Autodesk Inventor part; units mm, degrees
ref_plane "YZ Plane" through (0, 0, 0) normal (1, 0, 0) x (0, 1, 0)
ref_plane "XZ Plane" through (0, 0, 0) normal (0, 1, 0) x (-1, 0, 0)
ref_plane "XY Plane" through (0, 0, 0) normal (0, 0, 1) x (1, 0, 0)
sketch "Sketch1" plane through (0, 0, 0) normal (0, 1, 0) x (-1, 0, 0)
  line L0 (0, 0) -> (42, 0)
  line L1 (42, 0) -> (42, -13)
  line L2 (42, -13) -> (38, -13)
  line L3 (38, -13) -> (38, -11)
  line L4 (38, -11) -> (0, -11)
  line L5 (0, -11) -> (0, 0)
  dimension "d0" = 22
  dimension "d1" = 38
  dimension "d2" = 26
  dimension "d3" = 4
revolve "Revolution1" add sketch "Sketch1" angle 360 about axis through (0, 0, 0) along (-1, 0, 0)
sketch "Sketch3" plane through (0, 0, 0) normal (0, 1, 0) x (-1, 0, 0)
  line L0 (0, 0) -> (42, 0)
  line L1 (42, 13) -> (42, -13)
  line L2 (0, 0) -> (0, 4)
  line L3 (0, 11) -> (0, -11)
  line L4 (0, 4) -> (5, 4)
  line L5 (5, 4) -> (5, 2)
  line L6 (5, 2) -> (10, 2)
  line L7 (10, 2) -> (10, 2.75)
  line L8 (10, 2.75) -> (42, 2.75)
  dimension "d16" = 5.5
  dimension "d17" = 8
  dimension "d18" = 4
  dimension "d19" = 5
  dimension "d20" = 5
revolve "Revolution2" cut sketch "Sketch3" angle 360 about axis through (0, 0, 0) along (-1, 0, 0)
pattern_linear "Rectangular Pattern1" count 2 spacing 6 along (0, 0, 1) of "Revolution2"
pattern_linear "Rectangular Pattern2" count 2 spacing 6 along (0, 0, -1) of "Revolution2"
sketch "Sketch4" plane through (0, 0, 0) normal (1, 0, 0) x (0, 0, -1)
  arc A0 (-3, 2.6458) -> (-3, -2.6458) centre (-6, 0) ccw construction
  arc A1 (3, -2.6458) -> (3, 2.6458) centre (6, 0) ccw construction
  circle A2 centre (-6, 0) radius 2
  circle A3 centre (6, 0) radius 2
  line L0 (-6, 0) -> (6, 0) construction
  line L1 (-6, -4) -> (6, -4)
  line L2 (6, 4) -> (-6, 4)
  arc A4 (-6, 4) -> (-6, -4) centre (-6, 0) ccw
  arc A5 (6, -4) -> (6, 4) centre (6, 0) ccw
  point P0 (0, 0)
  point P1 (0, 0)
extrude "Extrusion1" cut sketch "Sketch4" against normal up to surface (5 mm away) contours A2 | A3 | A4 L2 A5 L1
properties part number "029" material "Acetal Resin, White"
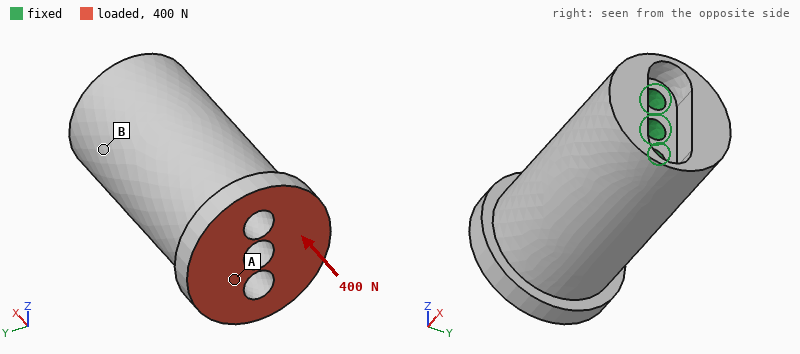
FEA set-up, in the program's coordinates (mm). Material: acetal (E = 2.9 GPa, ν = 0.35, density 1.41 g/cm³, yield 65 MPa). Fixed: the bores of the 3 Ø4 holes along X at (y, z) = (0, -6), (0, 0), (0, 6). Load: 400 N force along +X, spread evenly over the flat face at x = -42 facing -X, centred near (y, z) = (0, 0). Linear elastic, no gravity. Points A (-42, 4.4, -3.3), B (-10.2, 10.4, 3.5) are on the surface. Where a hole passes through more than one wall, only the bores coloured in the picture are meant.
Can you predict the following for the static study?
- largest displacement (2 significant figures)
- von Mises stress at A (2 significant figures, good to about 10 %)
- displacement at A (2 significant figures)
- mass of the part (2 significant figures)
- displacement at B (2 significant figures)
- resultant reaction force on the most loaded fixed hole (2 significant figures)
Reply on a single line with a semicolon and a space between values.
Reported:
23 µm; 1.4 MPa; 19 µm; 19 g; 9.2 µm; 140 N
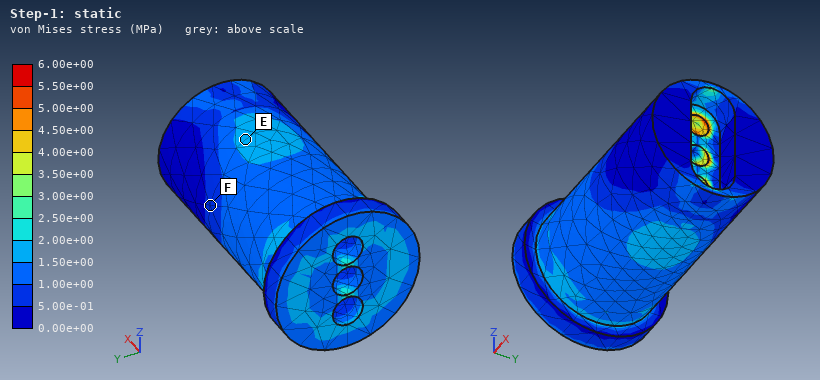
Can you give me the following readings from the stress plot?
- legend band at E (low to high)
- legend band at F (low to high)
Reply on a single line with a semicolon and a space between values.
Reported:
1.50e+00 to 2.00e+00 MPa; 5.00e-01 to 1.00e+00 MPa
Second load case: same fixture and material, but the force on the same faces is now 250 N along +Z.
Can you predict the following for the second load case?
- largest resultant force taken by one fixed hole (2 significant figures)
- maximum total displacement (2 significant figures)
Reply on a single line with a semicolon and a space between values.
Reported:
540 N; 0.25 mm
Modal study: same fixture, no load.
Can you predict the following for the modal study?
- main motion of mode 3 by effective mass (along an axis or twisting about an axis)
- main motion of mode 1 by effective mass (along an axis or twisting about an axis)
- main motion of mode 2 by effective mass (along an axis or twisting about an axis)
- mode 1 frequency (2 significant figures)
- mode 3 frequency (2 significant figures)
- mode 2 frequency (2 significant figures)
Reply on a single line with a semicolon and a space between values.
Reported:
twisting about X; along Y; along Z; 1400 Hz; 4900 Hz; 2200 Hz
